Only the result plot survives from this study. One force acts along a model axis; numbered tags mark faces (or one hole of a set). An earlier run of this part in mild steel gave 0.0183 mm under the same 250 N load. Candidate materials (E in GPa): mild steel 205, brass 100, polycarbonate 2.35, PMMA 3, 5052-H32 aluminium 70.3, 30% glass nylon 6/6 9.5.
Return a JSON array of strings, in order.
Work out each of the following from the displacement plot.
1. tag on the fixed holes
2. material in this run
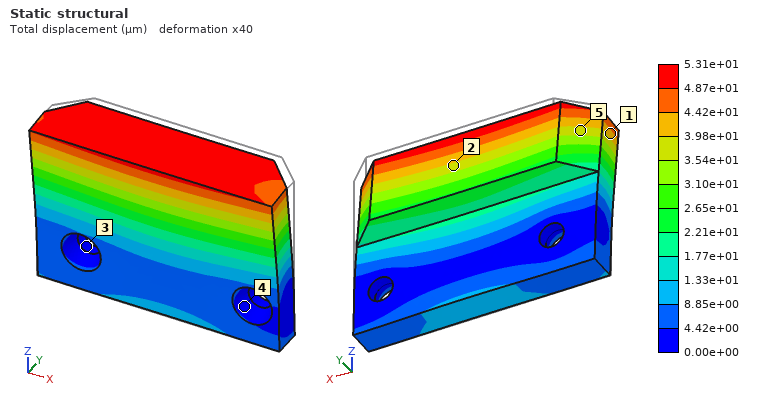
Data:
["3", "5052-H32 aluminium"]
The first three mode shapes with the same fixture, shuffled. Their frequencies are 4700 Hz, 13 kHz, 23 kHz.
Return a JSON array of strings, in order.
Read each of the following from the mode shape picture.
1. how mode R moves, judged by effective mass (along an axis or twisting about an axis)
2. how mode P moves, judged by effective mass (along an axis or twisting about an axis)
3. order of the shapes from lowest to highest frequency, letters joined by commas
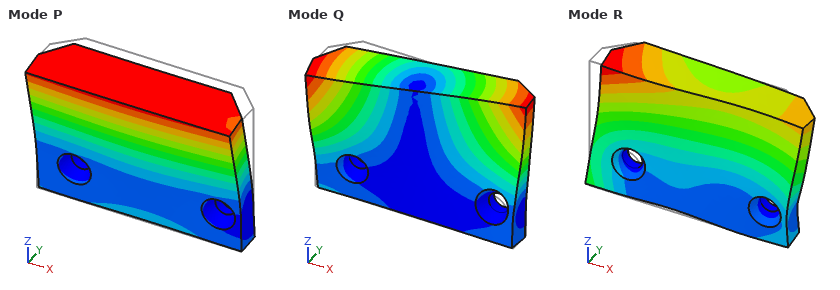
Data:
["along X", "along Y", "P, Q, R"]
